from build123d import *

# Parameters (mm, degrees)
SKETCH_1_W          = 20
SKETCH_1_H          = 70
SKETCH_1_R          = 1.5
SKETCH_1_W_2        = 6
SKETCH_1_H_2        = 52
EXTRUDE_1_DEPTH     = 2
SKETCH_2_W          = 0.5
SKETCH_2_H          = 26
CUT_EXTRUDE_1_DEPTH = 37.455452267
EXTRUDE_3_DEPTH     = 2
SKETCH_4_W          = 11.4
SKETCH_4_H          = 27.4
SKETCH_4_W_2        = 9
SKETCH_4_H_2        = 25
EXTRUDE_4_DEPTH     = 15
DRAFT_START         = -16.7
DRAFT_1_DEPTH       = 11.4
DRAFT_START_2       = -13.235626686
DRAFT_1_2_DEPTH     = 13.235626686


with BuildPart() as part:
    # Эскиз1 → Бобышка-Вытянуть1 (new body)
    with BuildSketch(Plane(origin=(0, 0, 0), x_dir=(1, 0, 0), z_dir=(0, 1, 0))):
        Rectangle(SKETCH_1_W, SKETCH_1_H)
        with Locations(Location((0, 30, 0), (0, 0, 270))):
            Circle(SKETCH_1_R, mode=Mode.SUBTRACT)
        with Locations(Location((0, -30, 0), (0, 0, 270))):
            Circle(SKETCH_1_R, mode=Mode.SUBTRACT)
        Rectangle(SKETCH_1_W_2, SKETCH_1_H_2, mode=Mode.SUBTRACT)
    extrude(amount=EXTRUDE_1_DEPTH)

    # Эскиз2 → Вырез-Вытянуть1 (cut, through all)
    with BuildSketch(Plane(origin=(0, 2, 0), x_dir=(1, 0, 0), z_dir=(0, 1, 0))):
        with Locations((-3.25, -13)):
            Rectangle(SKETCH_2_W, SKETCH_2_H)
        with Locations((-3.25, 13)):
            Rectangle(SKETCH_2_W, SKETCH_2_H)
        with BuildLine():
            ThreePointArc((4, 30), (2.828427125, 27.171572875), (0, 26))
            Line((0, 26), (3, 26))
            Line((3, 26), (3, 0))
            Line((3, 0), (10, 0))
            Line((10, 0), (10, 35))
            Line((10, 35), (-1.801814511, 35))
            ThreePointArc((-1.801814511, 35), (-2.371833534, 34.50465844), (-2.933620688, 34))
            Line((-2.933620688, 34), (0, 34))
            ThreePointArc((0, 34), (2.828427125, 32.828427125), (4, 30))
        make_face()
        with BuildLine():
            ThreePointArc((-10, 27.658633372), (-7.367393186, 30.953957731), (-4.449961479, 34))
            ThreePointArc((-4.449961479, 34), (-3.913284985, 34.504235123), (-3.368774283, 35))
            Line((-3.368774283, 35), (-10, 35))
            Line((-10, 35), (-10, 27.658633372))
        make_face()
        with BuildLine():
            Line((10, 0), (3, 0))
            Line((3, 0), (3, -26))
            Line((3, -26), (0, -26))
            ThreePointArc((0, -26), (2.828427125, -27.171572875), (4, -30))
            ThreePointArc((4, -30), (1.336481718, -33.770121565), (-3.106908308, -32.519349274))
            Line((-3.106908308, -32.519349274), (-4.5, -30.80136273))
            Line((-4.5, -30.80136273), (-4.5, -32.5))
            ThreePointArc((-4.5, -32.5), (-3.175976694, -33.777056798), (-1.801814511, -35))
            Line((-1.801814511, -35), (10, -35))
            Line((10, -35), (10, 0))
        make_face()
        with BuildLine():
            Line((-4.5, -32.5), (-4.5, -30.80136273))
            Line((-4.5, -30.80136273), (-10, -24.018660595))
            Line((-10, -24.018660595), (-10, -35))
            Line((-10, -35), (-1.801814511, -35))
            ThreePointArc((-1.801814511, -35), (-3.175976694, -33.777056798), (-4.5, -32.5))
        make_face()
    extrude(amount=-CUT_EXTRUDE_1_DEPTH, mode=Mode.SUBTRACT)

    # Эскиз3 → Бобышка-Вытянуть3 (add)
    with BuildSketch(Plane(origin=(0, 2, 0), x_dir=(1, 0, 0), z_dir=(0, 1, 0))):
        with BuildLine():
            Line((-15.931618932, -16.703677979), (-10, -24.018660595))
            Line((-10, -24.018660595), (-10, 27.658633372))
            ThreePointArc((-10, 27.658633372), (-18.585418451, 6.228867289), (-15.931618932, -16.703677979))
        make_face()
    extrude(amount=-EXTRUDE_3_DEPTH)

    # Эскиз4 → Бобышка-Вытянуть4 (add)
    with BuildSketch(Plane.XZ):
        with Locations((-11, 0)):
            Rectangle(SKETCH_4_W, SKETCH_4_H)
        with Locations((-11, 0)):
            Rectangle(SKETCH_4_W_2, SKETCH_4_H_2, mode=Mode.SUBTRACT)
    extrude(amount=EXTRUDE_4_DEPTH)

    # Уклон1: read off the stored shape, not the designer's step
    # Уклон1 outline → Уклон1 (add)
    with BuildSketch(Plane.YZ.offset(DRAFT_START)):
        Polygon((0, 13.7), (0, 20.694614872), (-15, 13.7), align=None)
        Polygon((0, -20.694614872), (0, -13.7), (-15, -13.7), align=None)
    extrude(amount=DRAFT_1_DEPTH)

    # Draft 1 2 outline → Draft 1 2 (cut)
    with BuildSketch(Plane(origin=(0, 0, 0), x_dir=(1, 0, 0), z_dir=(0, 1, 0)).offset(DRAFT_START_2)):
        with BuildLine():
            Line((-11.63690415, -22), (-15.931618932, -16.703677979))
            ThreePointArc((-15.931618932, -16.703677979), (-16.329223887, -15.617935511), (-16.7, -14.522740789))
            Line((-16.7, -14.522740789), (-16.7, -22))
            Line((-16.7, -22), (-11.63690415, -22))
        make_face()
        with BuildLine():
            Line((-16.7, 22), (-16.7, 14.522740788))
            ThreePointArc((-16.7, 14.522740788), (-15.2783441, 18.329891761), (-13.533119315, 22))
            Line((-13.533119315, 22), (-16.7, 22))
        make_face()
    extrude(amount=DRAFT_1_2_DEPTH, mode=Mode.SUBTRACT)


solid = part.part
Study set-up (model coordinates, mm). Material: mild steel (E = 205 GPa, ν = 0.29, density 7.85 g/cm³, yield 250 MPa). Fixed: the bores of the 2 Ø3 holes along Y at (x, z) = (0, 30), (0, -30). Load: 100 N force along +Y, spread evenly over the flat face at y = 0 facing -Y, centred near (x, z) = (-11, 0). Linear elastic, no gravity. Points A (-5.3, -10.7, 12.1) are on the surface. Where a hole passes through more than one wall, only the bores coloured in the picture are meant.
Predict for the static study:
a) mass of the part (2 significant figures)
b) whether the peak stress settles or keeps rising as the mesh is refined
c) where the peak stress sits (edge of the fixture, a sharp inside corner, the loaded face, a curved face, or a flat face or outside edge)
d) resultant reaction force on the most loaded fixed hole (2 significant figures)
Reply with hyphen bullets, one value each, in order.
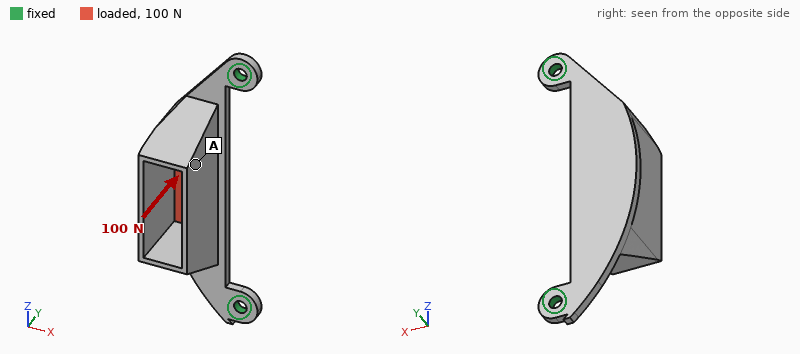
- 32 g
- keeps rising
- edge of the fixture
- 52 N
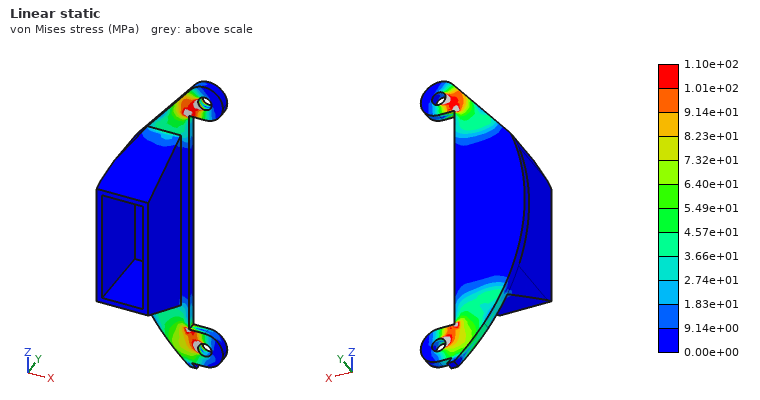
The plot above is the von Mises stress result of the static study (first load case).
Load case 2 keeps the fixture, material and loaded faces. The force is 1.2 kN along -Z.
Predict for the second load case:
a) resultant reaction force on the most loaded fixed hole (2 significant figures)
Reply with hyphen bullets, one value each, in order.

- 640 N
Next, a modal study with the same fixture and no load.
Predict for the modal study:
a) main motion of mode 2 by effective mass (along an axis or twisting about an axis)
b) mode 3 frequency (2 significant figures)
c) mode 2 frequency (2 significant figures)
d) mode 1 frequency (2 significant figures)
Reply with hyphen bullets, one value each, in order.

- along Y
- 4900 Hz
- 3800 Hz
- 1200 Hz
